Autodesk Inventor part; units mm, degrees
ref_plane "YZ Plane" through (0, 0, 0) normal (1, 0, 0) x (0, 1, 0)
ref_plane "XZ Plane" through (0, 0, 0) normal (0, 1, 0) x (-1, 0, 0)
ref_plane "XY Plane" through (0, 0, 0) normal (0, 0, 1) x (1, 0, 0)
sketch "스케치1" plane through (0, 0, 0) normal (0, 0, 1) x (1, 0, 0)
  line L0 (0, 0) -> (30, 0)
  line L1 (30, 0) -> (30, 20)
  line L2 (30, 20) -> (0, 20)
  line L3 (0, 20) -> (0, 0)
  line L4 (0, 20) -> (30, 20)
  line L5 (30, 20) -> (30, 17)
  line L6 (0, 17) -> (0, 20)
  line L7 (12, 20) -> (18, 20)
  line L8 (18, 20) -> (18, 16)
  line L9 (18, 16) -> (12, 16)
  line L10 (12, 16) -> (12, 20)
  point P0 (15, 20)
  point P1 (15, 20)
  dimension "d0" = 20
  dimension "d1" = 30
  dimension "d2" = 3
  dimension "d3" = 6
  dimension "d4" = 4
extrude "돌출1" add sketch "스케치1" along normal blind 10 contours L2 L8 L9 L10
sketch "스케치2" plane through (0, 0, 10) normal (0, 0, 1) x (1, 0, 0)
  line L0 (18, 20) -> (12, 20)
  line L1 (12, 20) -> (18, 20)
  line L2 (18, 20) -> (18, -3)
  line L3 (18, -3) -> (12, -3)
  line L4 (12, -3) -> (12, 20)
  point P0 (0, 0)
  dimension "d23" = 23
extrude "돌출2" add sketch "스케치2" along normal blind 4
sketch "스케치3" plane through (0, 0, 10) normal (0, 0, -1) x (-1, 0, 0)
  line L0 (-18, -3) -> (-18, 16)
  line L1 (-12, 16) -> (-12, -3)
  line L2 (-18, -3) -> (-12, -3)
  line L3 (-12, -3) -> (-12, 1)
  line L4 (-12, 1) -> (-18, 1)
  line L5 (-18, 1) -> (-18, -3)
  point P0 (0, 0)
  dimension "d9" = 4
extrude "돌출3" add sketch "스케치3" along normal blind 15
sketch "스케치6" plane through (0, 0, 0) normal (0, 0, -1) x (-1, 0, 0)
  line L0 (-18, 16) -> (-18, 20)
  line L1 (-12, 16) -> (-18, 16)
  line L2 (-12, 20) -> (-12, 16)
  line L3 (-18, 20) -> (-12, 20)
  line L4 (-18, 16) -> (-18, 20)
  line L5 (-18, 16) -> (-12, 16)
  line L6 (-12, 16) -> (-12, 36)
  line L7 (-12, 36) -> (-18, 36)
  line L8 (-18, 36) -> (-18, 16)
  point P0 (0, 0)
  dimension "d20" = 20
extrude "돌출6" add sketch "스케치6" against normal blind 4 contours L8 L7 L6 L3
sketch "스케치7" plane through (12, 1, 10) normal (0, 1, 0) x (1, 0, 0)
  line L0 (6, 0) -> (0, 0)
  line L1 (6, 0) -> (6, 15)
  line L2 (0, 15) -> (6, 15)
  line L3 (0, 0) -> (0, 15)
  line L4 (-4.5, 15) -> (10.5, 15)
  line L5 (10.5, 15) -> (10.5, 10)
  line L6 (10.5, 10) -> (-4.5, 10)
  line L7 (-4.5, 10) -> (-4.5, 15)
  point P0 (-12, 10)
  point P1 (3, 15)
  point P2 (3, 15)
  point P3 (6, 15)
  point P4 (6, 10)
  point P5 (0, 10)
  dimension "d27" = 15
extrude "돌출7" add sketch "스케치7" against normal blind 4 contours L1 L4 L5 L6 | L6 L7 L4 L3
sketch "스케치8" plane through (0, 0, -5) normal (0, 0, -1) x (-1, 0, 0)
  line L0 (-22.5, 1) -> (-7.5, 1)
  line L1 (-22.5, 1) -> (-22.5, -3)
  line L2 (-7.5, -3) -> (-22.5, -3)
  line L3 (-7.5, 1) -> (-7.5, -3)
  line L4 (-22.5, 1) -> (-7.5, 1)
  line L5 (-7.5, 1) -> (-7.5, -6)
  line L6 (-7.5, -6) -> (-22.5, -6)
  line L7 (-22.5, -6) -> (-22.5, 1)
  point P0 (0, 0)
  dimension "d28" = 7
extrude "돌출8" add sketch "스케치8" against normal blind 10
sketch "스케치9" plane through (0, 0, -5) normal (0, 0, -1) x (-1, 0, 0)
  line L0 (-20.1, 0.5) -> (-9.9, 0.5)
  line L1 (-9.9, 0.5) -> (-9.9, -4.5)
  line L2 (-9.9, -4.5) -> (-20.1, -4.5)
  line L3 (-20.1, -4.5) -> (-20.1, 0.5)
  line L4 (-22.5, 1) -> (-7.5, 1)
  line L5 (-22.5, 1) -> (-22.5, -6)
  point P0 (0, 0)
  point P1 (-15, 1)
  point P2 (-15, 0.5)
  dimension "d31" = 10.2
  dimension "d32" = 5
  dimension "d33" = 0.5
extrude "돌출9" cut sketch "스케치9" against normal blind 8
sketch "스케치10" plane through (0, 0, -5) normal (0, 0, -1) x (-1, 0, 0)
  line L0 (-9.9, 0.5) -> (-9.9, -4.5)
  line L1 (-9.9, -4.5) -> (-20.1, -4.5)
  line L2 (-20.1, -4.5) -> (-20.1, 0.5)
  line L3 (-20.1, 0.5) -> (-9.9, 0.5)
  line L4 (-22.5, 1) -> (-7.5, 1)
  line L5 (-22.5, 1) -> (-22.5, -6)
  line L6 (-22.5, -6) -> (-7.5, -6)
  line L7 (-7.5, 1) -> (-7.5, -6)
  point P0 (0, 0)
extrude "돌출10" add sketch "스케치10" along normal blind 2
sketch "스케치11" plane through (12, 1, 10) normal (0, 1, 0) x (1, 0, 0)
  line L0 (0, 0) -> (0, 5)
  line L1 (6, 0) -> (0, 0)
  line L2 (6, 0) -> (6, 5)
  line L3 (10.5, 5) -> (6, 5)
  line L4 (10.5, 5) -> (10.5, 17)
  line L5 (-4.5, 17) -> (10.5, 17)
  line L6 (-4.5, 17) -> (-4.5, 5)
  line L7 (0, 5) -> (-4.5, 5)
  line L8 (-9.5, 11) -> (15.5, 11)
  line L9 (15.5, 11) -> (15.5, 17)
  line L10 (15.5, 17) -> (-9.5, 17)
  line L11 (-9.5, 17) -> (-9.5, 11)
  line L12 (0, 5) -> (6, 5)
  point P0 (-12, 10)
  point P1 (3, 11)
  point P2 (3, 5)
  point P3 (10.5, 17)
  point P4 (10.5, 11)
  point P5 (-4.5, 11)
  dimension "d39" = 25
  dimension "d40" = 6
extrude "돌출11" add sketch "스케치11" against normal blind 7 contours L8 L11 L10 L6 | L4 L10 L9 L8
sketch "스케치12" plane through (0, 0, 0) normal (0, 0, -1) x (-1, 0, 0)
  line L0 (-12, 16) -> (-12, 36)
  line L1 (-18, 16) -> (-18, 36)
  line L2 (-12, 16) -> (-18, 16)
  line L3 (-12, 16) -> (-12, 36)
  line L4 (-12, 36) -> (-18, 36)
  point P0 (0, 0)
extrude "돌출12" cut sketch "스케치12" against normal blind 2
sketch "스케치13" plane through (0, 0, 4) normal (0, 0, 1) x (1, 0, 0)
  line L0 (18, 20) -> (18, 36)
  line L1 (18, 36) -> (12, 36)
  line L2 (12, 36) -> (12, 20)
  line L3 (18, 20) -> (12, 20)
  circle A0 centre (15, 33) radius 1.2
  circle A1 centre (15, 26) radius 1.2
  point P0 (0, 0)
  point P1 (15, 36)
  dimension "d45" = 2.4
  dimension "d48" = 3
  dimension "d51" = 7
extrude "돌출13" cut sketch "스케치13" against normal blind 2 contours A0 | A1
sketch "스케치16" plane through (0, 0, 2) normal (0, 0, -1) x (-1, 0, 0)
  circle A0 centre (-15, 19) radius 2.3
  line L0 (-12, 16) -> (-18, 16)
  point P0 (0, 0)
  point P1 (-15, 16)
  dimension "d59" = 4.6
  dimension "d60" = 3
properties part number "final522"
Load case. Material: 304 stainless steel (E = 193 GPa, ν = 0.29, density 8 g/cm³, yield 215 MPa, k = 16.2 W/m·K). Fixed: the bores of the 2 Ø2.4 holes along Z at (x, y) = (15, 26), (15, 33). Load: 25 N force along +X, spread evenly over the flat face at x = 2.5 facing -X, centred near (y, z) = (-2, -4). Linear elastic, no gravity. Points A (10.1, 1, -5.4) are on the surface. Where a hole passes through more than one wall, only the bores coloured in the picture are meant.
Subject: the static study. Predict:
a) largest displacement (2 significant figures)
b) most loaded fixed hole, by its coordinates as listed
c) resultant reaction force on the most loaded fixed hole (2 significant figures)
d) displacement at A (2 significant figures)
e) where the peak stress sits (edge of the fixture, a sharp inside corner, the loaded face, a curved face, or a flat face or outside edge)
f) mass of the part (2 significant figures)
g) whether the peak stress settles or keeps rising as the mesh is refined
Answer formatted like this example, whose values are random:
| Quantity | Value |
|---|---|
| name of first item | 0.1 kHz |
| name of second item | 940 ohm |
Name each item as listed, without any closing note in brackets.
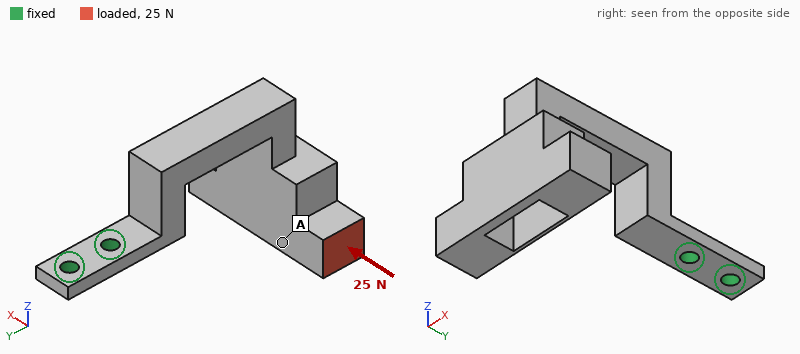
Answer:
| Quantity | Value |
|---|---|
| largest displacement | 94 µm |
| most loaded fixed hole, by its coordinates as listed | (15, 26) |
| resultant reaction force on the most loaded fixed hole | 59 N |
| displacement at A | 70 µm |
| where the peak stress sits | edge of the fixture |
| mass of the part | 18 g |
| whether the peak stress settles or keeps rising as the mesh is refined | keeps rising |
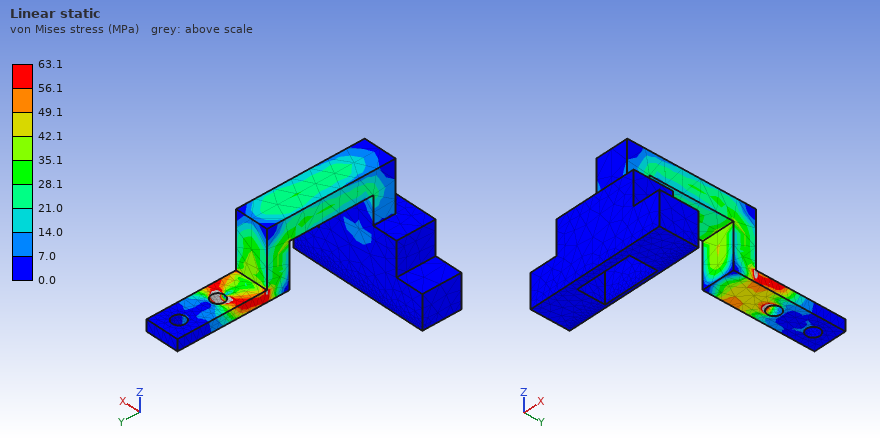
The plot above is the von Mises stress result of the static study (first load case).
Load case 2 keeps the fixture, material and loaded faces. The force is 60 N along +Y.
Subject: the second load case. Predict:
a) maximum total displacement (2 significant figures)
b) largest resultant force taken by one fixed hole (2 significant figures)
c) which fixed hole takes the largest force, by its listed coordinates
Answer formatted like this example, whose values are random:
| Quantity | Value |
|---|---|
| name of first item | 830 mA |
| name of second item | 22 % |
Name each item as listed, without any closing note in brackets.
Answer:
| Quantity | Value |
|---|---|
| maximum total displacement | 0.24 mm |
| largest resultant force taken by one fixed hole | 67 N |
| which fixed hole takes the largest force, by its listed coordinates | (15, 26) |
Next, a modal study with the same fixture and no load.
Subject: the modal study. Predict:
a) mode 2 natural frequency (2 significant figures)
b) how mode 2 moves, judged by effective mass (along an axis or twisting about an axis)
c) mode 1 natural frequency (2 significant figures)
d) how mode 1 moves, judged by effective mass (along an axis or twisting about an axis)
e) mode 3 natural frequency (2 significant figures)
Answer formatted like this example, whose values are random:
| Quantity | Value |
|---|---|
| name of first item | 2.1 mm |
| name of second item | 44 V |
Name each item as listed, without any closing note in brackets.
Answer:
| Quantity | Value |
|---|---|
| mode 2 natural frequency | 960 Hz |
| how mode 2 moves, judged by effective mass | along X |
| mode 1 natural frequency | 560 Hz |
| how mode 1 moves, judged by effective mass | along Z |
| mode 3 natural frequency | 1800 Hz |
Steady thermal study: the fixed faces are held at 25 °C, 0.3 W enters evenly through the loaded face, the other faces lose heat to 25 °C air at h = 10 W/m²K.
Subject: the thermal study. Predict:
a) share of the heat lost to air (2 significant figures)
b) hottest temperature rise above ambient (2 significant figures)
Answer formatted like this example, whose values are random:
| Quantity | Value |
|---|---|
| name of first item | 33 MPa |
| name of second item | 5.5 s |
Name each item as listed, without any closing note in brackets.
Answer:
| Quantity | Value |
|---|---|
| share of the heat lost to air | 71 % |
| hottest temperature rise above ambient | 19 K |
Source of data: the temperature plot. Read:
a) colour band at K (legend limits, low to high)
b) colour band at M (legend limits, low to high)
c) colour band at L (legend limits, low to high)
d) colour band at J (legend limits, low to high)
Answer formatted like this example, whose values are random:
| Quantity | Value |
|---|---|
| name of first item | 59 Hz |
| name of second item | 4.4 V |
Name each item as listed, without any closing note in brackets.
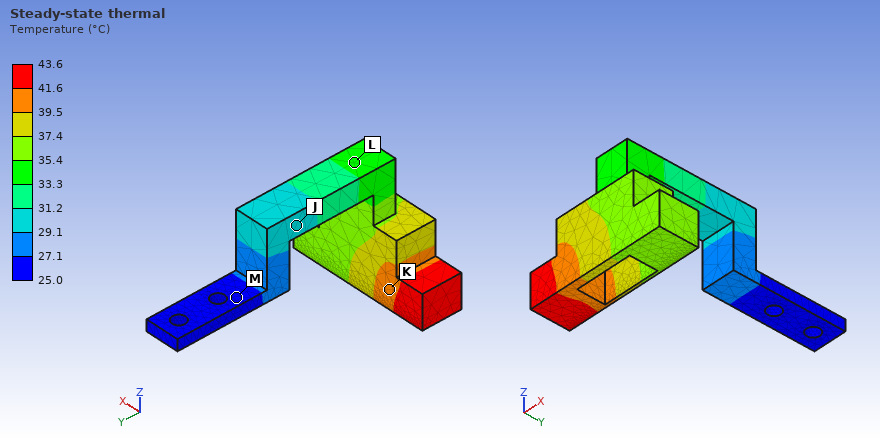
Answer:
| Quantity | Value |
|---|---|
| colour band at K | 39.5 to 41.6 °C |
| colour band at M | 25.0 to 27.1 °C |
| colour band at L | 33.3 to 35.4 °C |
| colour band at J | 29.1 to 31.2 °C |
